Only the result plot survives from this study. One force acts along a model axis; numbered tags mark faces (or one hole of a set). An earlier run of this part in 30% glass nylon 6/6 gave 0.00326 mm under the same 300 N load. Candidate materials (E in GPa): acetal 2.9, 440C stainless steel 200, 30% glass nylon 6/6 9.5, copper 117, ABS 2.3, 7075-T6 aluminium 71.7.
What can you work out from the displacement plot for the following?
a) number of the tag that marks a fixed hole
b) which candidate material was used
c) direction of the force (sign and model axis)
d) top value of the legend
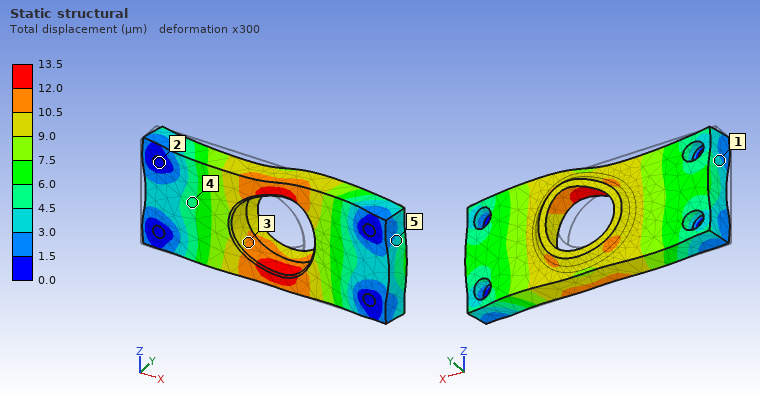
2
ABS
+X
13.5 µm
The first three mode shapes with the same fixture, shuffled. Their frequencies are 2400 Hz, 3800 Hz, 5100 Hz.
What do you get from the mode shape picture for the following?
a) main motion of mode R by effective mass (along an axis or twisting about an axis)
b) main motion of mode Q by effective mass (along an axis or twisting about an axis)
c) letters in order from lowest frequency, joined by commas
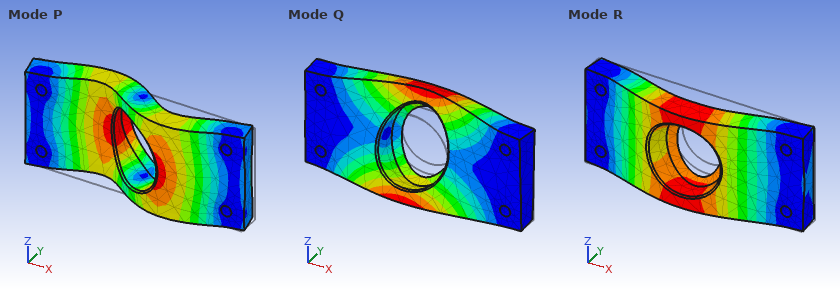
along Y
twisting about X
R, Q, P
